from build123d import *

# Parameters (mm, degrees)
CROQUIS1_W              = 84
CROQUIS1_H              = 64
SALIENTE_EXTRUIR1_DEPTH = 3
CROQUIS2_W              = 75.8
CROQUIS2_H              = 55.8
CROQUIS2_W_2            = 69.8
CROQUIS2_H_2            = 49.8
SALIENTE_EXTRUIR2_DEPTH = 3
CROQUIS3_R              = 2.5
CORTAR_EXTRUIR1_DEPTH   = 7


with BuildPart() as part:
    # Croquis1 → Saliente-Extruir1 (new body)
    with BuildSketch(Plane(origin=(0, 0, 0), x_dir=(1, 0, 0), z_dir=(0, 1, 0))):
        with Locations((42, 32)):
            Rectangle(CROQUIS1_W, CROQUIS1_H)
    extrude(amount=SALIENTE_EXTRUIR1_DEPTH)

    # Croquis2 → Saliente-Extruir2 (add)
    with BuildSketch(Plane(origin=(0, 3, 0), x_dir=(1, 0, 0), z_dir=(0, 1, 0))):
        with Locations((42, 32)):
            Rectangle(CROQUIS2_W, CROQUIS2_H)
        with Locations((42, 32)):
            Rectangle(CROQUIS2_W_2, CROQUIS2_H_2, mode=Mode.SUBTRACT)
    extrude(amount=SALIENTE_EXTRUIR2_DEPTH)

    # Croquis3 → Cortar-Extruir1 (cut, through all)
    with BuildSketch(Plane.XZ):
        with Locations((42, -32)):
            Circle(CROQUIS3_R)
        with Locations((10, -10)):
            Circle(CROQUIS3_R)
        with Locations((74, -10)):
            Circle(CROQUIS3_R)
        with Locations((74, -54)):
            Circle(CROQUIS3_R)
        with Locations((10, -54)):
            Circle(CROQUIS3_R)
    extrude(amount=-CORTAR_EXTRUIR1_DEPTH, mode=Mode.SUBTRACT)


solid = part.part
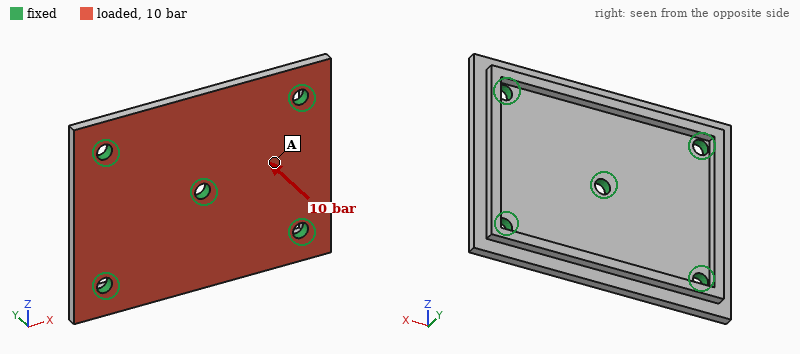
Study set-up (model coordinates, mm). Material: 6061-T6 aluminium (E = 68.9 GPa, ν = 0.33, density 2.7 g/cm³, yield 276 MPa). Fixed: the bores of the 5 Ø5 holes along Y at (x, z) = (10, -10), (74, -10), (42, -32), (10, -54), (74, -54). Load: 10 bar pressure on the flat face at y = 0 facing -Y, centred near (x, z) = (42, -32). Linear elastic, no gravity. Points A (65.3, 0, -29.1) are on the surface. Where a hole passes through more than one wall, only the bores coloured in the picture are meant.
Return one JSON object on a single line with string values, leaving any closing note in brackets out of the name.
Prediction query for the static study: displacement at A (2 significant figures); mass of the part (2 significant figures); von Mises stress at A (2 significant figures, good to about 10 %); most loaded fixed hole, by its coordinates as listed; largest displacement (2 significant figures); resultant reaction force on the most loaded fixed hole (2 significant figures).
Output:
{"displacement at A": "0.035 mm", "mass of the part": "49 g", "von Mises stress at A": "22 MPa", "most loaded fixed hole, by its coordinates as listed": "(42, -32)", "largest displacement": "0.11 mm", "resultant reaction force on the most loaded fixed hole": "1.4 kN"}
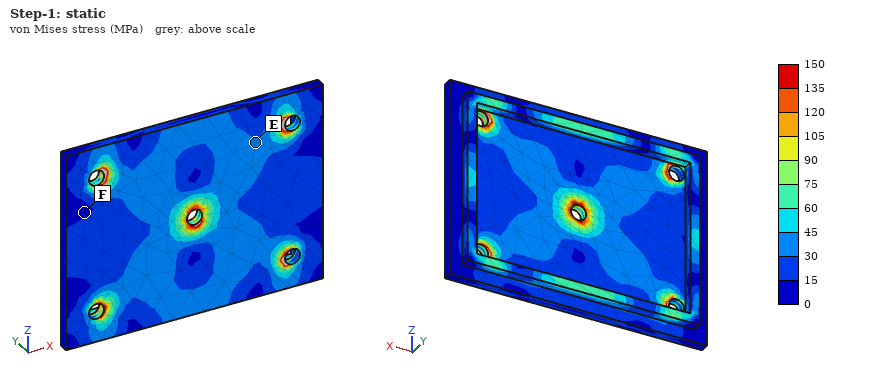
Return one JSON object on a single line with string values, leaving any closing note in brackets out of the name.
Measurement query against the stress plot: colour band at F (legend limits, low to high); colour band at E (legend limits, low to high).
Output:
{"colour band at F": "0 to 15 MPa", "colour band at E": "30 to 45 MPa"}
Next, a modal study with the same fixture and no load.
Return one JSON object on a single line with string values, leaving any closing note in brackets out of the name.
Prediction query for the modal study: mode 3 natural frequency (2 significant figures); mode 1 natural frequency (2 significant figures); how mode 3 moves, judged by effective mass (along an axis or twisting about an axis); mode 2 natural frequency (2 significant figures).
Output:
{"mode 3 natural frequency": "10 kHz", "mode 1 natural frequency": "6200 Hz", "how mode 3 moves, judged by effective mass": "twisting about Z", "mode 2 natural frequency": "6300 Hz"}
